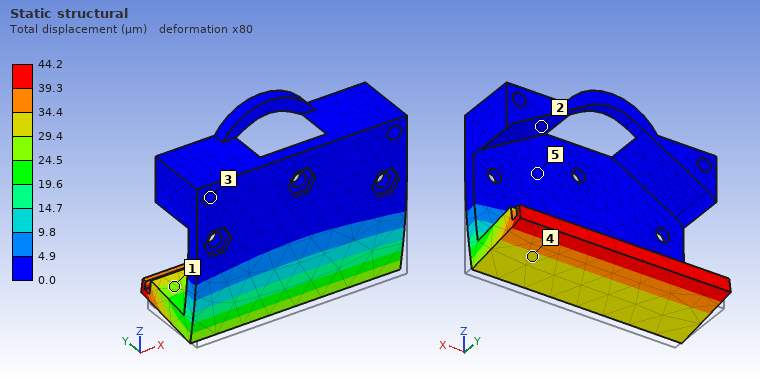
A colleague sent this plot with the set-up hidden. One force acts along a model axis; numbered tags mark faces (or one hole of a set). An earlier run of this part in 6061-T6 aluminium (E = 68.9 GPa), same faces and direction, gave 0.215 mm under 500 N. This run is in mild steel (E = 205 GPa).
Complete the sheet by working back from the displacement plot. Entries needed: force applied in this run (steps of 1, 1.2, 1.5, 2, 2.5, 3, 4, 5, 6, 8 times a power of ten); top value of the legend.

300 N
44.2 µm
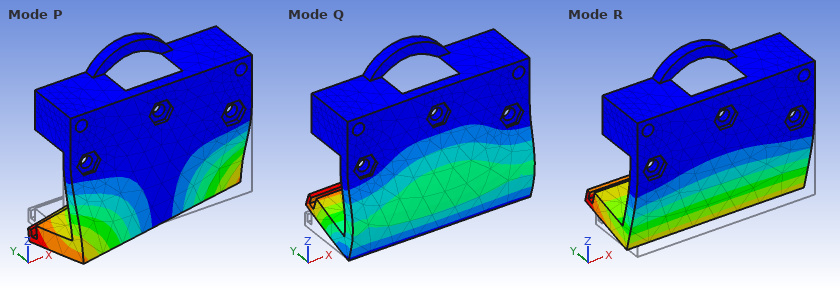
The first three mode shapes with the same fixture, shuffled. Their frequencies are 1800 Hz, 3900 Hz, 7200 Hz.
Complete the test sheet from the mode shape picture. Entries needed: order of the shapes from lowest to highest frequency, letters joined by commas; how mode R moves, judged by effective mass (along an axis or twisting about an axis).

R, P, Q
along Y
